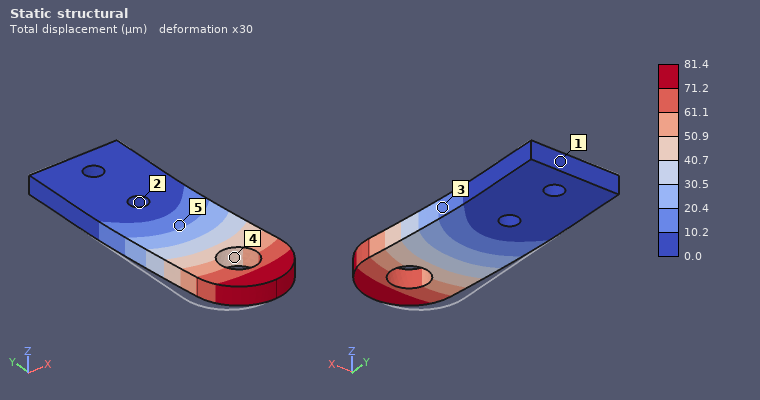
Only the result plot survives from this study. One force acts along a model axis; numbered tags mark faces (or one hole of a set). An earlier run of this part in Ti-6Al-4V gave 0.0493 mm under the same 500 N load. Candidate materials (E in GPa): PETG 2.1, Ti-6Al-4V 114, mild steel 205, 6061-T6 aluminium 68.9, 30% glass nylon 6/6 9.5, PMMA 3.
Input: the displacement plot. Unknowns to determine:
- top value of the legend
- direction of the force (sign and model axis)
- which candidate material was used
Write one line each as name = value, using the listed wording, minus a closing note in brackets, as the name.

top value of the legend = 81.4 µm
direction of the force = +X
which candidate material was used = 6061-T6 aluminium
